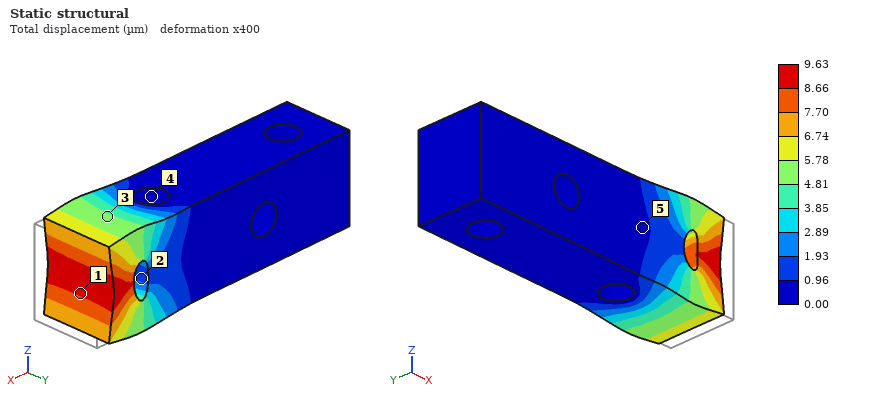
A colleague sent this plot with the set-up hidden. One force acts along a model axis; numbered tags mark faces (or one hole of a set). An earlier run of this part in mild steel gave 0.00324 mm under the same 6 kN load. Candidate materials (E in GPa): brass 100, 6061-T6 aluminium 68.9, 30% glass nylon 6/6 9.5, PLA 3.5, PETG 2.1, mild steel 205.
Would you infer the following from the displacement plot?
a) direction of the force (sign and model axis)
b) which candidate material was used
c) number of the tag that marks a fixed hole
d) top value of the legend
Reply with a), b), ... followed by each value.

a) -X
b) 6061-T6 aluminium
c) 4
d) 9.63 µm
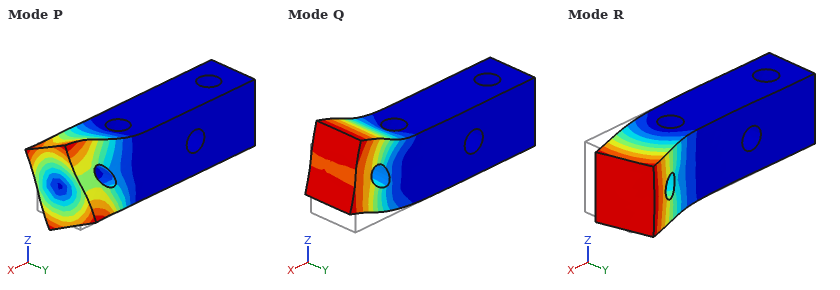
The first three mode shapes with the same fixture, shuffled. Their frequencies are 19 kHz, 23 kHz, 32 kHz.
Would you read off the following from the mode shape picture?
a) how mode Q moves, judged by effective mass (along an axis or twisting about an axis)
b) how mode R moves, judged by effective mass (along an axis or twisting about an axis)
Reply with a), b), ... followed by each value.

a) along Z
b) along Y
